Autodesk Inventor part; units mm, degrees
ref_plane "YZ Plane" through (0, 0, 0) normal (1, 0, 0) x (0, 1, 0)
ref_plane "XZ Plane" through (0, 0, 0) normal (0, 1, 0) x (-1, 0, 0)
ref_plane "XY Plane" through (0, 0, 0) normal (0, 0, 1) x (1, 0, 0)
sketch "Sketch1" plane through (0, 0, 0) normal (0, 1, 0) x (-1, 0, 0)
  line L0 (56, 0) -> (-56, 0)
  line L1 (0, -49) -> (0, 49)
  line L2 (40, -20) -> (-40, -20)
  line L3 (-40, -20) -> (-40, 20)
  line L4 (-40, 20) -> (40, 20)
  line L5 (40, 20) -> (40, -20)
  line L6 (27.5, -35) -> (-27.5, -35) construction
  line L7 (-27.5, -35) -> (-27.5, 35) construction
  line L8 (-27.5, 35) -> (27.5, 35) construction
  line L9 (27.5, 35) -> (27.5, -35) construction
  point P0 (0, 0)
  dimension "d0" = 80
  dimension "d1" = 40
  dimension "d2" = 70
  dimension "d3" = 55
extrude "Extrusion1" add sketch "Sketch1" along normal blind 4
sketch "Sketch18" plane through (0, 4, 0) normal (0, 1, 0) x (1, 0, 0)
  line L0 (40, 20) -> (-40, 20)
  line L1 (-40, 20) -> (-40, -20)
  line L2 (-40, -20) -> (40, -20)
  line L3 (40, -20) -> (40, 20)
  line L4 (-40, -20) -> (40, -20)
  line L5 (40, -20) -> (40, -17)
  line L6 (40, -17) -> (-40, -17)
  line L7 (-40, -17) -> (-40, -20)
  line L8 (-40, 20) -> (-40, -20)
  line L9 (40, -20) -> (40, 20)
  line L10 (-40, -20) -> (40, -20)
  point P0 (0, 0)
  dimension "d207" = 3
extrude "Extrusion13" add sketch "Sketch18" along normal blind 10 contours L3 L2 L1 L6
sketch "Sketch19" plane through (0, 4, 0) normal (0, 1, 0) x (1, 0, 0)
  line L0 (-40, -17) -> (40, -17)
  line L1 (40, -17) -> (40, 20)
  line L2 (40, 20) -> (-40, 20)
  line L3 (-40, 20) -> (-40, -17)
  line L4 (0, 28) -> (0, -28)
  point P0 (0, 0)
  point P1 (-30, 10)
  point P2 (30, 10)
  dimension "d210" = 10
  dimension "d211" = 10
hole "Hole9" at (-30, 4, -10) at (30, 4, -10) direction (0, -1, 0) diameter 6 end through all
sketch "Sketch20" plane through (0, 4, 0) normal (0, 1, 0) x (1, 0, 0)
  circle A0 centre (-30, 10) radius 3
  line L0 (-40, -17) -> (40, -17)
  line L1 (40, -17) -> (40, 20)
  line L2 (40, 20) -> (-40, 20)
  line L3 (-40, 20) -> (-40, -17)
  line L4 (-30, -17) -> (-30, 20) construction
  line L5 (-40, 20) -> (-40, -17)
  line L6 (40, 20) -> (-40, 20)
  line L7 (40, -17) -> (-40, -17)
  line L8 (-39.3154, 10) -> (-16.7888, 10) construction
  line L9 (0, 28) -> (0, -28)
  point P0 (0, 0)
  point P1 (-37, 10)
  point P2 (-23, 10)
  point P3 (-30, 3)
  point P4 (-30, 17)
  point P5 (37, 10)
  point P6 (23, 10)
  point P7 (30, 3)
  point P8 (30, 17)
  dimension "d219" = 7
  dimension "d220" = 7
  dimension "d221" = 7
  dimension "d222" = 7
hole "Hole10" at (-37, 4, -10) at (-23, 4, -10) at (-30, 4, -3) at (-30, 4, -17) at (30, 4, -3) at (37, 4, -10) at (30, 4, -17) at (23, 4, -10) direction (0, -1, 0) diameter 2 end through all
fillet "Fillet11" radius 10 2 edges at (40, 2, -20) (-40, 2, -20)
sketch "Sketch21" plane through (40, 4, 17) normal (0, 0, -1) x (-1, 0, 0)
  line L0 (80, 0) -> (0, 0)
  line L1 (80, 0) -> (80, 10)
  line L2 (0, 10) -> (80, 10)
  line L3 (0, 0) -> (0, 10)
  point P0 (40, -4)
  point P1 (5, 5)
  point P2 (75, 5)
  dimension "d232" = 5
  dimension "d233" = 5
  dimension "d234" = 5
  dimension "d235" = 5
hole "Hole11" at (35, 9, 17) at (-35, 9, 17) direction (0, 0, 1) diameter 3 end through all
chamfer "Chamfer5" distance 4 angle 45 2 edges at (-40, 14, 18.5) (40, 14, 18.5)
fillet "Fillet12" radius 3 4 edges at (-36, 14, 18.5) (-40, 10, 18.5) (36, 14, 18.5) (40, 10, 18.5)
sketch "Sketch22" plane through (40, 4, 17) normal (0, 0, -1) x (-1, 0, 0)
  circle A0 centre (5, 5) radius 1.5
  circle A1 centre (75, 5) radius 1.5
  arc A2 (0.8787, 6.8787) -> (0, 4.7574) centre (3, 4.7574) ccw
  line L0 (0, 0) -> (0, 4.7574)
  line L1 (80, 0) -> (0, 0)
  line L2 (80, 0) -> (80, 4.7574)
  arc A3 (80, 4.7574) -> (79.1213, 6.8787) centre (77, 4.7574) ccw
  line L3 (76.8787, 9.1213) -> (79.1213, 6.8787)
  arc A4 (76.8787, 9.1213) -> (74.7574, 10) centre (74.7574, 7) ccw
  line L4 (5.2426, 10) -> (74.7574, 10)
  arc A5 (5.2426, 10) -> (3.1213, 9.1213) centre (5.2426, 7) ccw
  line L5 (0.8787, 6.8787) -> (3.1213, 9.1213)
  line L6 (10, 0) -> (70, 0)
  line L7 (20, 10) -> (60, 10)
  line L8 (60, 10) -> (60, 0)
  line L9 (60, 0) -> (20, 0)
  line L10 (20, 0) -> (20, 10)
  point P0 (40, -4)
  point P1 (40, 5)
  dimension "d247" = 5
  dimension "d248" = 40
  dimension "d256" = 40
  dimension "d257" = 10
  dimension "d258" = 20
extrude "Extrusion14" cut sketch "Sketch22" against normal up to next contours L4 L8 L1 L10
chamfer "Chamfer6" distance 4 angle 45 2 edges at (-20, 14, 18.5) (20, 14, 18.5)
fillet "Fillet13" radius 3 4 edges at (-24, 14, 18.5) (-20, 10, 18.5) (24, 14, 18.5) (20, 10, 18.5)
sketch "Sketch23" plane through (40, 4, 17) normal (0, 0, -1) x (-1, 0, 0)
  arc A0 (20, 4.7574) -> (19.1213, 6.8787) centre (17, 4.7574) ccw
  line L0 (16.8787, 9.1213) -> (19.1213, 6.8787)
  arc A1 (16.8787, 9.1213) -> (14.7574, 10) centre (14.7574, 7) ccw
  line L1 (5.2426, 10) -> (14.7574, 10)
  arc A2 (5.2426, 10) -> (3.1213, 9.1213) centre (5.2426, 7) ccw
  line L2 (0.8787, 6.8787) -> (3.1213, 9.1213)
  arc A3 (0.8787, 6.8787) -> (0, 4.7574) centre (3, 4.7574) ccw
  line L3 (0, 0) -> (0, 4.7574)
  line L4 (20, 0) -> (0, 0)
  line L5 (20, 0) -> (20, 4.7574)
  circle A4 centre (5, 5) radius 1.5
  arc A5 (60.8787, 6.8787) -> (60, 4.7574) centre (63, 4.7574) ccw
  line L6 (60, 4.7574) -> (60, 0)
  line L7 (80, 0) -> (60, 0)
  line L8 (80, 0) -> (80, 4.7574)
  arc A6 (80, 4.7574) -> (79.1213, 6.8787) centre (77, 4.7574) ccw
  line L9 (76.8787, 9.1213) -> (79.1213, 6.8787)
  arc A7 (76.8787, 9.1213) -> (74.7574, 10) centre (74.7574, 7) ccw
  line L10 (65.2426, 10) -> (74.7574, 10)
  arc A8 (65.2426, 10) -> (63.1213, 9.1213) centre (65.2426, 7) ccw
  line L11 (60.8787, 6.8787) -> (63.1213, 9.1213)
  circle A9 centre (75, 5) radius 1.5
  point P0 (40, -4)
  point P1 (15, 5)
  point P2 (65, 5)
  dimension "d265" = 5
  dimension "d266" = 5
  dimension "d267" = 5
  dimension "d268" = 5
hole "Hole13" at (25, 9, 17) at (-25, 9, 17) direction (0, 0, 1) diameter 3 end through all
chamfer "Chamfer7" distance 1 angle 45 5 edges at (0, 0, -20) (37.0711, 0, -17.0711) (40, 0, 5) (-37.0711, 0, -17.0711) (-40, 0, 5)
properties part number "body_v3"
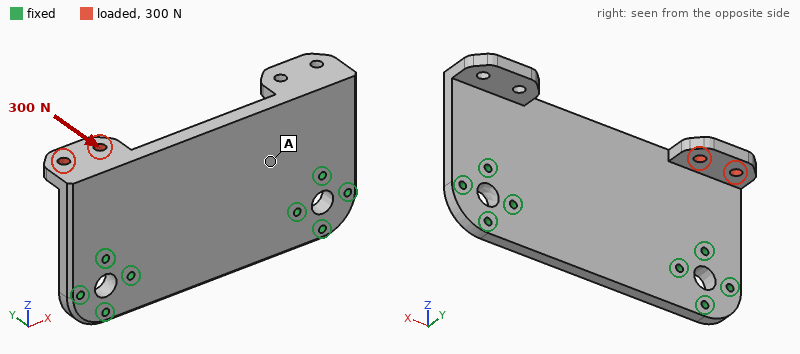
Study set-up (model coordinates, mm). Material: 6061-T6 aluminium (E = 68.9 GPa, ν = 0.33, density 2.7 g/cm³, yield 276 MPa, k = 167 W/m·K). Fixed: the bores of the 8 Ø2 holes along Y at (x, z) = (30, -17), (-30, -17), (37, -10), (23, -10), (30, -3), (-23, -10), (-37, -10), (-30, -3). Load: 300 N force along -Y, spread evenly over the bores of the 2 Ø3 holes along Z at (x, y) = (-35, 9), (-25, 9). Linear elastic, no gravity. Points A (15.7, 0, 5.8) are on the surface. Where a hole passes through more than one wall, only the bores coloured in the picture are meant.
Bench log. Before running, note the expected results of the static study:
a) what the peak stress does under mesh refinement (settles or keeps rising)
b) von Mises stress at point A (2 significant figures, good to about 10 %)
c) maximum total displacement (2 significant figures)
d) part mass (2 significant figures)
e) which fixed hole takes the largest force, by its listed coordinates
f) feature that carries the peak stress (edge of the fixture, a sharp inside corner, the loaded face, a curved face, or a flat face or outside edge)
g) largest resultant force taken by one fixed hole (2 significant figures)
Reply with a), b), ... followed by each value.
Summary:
a) keeps rising
b) 8.6 MPa
c) 0.15 mm
d) 36 g
e) (-30, -3)
f) edge of the fixture
g) 550 N
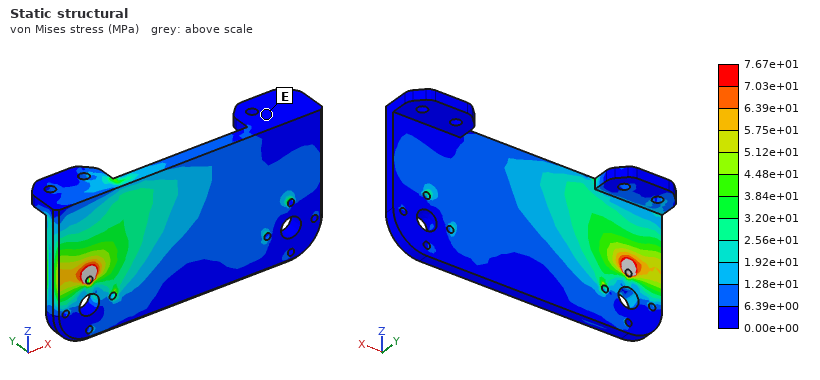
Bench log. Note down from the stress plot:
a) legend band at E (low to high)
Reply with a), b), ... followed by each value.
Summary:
a) 0.00e+00 to 6.39e+00 MPa
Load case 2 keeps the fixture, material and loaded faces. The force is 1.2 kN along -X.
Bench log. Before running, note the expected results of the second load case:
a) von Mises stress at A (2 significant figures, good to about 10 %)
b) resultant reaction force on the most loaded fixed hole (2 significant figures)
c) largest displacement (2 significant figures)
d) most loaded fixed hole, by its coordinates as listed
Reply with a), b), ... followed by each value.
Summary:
a) 16 MPa
b) 560 N
c) 0.17 mm
d) (-30, -3)
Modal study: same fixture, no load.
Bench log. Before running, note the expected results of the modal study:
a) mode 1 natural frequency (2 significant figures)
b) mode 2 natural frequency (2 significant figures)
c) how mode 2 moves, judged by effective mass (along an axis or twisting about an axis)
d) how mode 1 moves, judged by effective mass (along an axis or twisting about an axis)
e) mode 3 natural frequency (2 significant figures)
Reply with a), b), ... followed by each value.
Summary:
a) 3400 Hz
b) 4800 Hz
c) twisting about Z
d) along Y
e) 6100 Hz
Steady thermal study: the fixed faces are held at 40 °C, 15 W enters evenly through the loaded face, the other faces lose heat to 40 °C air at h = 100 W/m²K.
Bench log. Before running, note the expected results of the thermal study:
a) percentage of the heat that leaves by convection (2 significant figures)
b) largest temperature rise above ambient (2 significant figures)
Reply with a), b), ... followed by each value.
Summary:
a) 21 %
b) 28 K
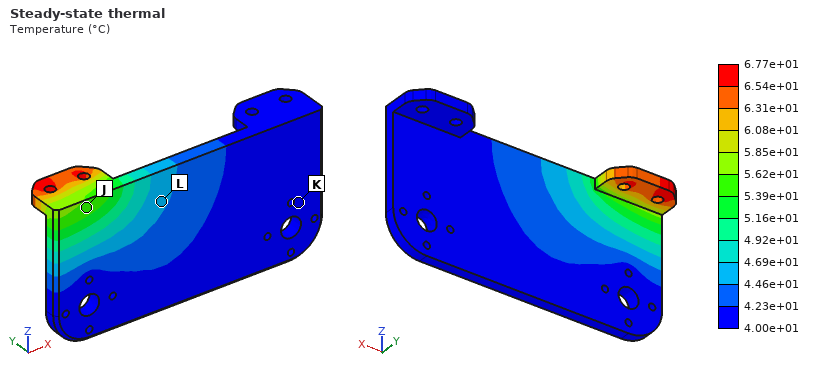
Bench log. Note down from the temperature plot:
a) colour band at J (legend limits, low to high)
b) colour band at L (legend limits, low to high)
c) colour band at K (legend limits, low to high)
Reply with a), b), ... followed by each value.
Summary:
a) 5.39e+01 to 5.62e+01 °C
b) 4.46e+01 to 4.69e+01 °C
c) 4.00e+01 to 4.23e+01 °C
